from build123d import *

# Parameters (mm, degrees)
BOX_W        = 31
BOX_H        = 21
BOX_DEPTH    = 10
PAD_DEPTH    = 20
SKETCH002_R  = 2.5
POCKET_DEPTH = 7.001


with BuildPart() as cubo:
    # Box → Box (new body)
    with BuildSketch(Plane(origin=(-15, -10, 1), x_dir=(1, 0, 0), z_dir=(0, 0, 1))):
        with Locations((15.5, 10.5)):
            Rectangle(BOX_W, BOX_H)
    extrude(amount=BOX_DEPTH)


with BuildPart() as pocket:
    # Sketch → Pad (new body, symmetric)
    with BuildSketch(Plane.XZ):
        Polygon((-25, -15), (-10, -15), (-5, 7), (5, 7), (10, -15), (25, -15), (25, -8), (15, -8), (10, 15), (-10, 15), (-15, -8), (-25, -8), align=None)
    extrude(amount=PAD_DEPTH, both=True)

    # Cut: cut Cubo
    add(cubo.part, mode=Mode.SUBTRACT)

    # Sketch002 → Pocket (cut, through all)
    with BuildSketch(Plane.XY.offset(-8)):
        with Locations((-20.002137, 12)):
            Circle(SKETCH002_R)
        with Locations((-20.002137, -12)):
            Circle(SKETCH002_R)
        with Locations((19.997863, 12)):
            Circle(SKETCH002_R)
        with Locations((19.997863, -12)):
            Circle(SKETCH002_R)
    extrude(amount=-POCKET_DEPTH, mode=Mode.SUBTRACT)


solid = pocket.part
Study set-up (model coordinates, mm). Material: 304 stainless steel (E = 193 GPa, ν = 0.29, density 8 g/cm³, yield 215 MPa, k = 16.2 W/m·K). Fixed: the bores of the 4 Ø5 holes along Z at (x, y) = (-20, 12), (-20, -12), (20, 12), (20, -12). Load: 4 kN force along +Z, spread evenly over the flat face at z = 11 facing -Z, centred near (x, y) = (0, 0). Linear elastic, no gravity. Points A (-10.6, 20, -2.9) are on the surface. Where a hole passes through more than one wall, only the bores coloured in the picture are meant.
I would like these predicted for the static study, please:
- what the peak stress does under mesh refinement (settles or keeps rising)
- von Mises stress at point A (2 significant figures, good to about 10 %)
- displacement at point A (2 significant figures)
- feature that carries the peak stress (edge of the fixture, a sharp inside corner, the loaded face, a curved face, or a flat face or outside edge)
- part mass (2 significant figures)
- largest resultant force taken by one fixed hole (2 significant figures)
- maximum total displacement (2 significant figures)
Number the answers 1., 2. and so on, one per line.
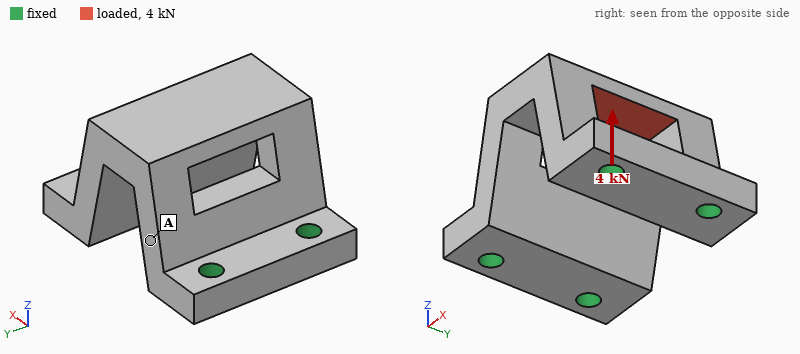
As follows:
1. keeps rising
2. 17 MPa
3. 3.3 µm
4. a sharp inside corner
5. 160 g
6. 1.1 kN
7. 19 µm
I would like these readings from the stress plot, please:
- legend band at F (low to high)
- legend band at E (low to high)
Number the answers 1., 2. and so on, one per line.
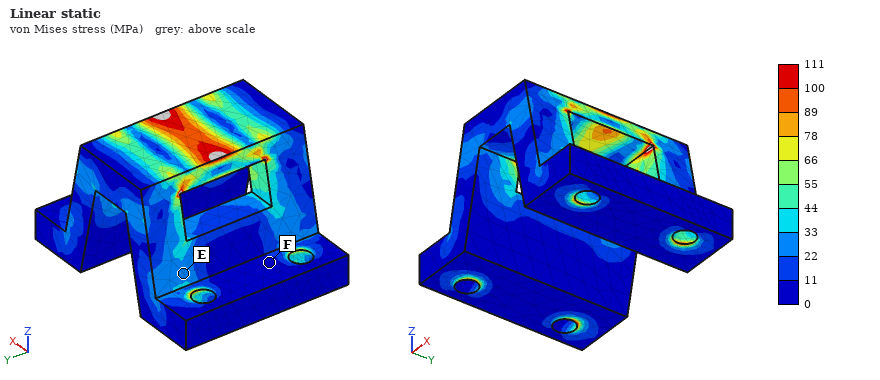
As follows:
1. 0 to 11 MPa
2. 22 to 33 MPa
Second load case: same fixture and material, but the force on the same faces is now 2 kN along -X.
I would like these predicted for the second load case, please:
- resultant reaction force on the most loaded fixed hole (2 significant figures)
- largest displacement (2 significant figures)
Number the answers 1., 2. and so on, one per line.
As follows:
1. 750 N
2. 11 µm
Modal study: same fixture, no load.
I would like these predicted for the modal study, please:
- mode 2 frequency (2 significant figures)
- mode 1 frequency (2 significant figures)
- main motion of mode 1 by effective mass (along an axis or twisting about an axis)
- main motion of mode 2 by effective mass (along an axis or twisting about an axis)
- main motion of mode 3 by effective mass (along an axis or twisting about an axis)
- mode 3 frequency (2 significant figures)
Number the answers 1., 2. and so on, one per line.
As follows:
1. 11 kHz
2. 9800 Hz
3. along Y
4. along X
5. twisting about Z
6. 14 kHz
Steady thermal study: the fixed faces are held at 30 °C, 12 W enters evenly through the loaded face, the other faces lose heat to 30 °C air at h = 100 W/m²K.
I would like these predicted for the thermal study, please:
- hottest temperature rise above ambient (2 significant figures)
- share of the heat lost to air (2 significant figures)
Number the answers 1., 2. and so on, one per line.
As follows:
1. 54 K
2. 74 %
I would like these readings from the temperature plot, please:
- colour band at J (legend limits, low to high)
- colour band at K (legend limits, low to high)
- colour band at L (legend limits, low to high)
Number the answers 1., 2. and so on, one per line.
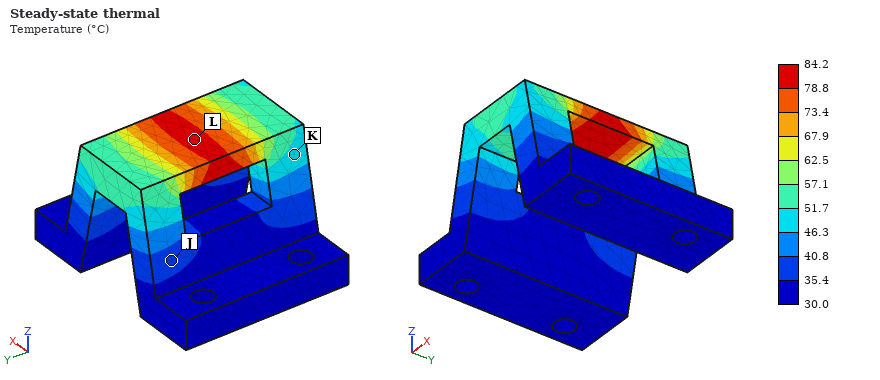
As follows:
1. 35.4 to 40.8 °C
2. 46.3 to 51.7 °C
3. 78.8 to 84.2 °C
